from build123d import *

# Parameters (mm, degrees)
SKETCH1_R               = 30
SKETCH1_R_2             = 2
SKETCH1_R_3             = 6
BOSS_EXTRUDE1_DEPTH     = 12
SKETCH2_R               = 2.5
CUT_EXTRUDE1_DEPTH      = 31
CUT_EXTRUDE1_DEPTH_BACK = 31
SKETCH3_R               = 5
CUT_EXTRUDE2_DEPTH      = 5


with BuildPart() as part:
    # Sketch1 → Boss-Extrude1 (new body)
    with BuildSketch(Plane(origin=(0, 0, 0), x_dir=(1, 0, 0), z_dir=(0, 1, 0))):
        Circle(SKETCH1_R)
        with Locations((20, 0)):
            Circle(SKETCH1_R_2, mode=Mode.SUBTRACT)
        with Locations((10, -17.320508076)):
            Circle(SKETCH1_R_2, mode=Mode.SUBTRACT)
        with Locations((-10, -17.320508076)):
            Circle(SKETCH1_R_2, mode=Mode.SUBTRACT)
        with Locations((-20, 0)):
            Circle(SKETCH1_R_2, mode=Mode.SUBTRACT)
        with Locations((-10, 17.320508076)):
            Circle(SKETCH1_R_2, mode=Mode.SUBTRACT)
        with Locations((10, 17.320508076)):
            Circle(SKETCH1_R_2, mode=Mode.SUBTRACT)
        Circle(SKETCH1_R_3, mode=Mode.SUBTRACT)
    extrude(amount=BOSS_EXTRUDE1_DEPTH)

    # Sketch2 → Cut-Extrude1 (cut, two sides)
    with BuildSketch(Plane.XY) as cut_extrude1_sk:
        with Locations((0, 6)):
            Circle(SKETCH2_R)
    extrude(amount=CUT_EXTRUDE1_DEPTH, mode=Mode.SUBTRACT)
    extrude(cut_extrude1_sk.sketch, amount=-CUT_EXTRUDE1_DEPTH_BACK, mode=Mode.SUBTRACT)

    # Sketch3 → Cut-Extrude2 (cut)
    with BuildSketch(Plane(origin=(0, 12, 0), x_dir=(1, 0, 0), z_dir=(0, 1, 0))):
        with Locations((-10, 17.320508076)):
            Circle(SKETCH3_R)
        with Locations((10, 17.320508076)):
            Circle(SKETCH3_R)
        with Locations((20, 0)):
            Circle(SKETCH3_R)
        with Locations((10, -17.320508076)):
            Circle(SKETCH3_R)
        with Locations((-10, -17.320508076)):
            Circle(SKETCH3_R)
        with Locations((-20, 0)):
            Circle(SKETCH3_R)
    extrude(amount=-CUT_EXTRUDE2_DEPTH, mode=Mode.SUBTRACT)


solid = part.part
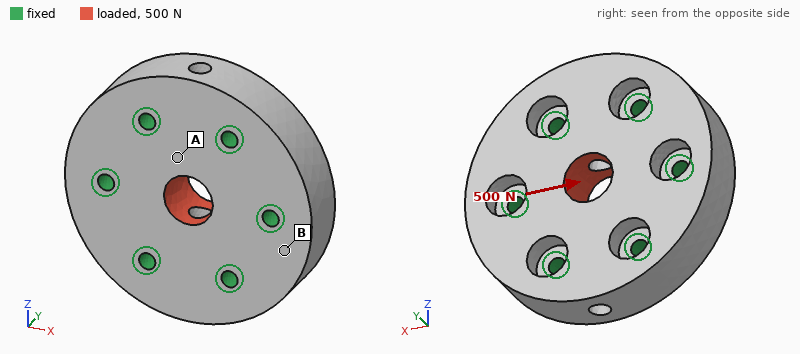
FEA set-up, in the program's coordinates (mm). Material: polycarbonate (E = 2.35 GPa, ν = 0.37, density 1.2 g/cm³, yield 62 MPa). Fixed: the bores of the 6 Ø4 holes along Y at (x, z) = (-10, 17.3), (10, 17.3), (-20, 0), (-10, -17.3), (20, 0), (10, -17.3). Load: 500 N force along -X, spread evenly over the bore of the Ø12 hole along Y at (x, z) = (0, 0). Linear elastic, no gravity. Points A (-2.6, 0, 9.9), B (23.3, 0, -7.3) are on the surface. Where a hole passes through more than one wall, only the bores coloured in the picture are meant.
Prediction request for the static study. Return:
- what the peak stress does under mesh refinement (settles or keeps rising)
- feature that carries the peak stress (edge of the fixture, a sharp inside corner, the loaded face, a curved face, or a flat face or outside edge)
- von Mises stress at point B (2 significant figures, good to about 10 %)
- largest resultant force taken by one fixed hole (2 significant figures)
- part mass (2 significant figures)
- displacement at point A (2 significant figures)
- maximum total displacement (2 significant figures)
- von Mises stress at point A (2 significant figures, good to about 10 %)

keeps rising
edge of the fixture
0.42 MPa
130 N
34 g
3.8 µm
11 µm
1.0 MPa
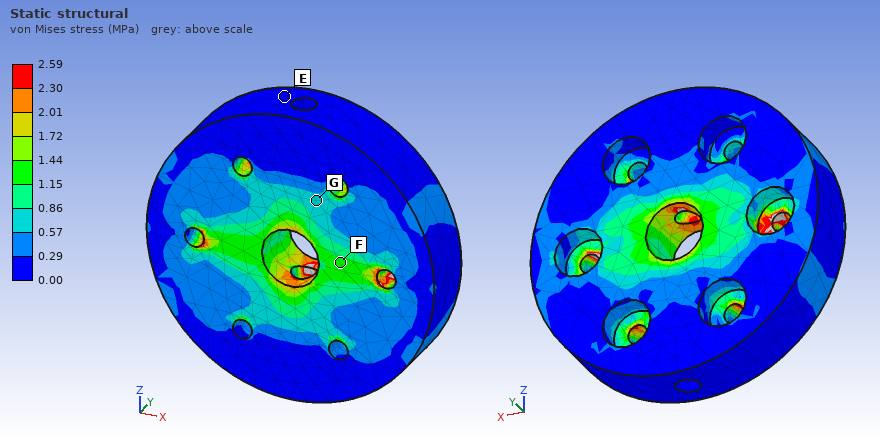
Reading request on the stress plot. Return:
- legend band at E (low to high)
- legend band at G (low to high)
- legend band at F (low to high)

0.00 to 0.29 MPa
0.57 to 0.86 MPa
1.15 to 1.44 MPa
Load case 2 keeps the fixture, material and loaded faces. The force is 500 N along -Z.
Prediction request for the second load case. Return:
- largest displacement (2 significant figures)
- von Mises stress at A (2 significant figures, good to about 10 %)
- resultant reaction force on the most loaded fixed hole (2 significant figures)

9.9 µm
1.0 MPa
110 N
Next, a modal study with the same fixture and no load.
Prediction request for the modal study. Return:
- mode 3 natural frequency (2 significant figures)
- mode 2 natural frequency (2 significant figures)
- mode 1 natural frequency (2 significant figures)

8200 Hz
8200 Hz
7900 Hz
